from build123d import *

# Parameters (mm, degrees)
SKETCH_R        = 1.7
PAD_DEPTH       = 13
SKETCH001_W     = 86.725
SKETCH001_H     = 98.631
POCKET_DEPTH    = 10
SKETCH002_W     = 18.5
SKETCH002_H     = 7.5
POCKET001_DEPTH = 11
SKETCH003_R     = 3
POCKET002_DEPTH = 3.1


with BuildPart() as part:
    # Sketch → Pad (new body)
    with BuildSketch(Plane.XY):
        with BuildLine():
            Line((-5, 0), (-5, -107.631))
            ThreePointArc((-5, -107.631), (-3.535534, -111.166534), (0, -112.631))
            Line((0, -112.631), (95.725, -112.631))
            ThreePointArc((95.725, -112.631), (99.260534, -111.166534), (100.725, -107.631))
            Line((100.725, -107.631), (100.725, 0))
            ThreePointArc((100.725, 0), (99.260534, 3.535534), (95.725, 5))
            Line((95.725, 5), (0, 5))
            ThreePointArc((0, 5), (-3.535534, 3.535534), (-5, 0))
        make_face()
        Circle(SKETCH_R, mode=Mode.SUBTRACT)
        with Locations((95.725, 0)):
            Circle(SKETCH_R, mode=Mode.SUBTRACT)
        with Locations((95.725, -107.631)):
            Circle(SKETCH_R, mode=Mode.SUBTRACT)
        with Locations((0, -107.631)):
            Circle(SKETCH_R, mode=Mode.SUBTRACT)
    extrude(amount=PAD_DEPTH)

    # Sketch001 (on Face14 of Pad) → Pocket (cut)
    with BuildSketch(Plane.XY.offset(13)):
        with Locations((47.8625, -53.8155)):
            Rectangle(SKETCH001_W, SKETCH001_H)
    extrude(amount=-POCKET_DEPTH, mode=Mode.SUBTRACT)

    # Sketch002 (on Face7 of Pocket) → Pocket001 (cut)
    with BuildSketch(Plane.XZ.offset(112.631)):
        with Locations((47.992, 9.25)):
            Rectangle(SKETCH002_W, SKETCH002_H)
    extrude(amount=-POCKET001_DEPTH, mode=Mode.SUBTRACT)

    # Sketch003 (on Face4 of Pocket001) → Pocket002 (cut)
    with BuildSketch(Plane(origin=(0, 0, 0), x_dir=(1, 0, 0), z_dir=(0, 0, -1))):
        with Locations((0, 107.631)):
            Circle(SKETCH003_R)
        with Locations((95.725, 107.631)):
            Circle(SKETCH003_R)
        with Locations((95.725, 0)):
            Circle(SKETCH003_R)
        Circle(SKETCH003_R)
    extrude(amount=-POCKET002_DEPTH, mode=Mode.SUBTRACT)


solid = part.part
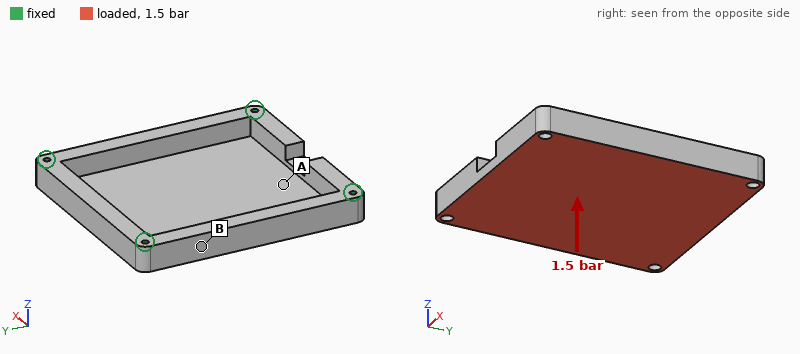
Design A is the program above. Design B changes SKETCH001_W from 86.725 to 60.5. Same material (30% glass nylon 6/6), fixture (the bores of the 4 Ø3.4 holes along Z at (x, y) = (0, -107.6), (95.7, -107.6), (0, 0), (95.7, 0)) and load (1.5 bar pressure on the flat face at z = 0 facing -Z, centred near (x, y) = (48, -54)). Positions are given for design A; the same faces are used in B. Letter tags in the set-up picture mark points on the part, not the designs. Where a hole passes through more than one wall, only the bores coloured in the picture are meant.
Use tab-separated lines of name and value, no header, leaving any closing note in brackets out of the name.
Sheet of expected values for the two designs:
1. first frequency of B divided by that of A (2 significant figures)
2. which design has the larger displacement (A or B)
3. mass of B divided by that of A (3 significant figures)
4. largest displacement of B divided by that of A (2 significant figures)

first frequency of B divided by that of A	1.4
which design has the larger displacement	A
mass of B divided by that of A	1.35
largest displacement of B divided by that of A	0.45
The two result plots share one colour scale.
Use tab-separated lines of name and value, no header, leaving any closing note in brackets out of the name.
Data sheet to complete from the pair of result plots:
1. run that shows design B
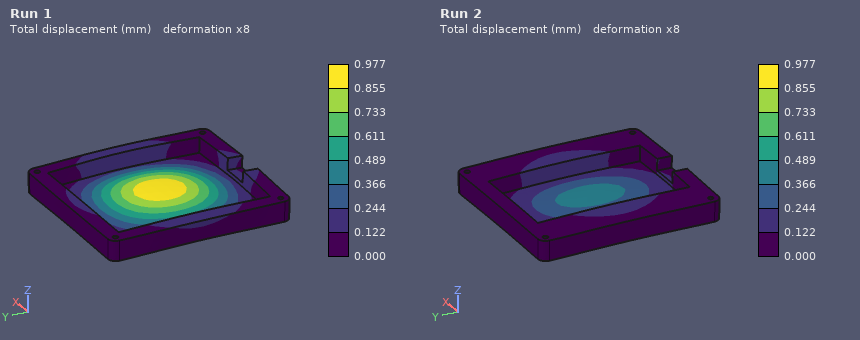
run that shows design B	Run 2
